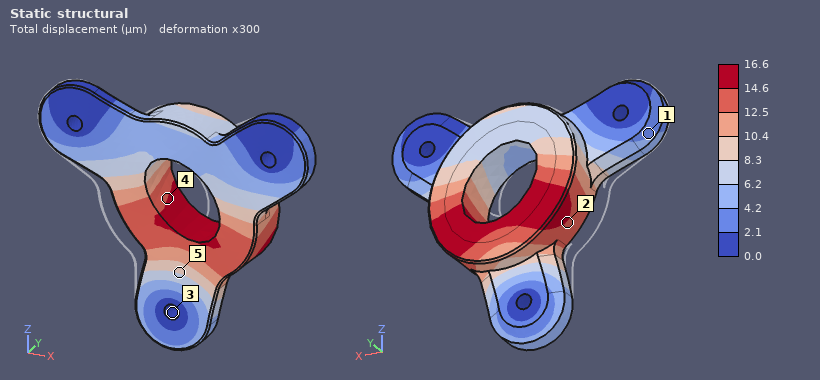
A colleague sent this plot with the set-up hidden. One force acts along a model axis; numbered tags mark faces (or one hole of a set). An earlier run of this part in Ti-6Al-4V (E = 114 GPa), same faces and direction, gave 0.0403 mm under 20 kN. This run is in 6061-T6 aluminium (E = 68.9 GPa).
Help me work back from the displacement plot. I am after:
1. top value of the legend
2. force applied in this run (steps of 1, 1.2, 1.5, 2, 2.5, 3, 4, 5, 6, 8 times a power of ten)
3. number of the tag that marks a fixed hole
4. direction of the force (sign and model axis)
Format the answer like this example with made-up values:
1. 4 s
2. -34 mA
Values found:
1. 16.6 µm
2. 5 kN
3. 3
4. +X
